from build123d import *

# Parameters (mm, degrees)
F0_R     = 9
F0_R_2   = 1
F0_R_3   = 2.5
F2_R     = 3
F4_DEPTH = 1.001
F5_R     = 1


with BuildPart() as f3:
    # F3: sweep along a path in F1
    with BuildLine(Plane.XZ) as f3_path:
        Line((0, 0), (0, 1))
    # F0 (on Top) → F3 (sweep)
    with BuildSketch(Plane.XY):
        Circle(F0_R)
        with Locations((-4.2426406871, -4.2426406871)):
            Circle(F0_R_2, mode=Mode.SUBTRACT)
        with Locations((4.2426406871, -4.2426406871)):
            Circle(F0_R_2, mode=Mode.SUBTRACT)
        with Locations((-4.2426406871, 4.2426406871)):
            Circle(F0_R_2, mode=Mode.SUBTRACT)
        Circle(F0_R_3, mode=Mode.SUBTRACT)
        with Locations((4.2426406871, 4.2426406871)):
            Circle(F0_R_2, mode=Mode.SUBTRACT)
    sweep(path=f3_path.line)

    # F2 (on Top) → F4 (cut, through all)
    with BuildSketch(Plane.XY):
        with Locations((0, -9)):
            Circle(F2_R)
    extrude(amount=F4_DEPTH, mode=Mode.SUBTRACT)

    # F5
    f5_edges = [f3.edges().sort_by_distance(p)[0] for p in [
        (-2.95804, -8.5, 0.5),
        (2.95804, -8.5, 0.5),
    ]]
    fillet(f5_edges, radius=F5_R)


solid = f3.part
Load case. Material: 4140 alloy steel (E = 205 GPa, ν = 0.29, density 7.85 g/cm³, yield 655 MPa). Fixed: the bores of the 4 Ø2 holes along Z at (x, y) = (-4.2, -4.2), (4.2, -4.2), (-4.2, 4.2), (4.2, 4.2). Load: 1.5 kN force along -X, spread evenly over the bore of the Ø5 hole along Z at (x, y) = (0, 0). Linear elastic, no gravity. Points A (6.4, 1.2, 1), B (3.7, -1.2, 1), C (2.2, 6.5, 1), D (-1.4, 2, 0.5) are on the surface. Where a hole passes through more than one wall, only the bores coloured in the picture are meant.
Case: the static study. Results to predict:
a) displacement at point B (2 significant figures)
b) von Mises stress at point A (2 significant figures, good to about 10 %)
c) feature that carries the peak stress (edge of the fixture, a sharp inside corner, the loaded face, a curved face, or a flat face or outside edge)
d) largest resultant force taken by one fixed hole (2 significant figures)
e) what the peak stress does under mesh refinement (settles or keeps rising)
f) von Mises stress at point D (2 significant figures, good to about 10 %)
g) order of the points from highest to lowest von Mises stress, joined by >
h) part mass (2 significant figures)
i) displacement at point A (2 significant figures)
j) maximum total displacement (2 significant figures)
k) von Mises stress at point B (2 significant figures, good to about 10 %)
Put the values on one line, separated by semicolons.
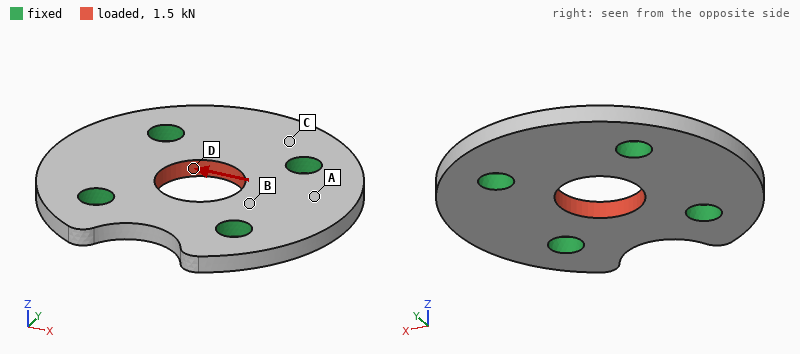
1.6 µm; 39 MPa; edge of the fixture; 390 N; keeps rising; 160 MPa; D > B > A > C; 1.6 g; 1.1 µm; 2.3 µm; 73 MPa
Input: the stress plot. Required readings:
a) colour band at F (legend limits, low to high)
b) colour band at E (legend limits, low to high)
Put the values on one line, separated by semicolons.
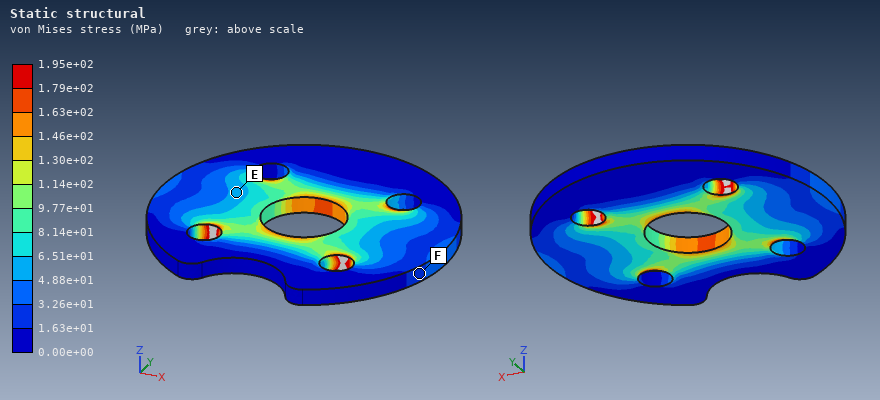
1.63e+01 to 3.26e+01 MPa; 4.88e+01 to 6.51e+01 MPa
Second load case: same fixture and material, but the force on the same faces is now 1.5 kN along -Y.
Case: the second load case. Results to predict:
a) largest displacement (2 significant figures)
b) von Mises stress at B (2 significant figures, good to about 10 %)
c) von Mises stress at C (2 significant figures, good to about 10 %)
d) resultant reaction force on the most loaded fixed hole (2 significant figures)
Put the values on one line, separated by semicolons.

2.8 µm; 82 MPa; 44 MPa; 400 N
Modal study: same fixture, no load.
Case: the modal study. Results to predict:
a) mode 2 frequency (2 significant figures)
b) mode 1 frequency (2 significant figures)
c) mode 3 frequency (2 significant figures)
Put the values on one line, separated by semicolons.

46 kHz; 45 kHz; 46 kHz
